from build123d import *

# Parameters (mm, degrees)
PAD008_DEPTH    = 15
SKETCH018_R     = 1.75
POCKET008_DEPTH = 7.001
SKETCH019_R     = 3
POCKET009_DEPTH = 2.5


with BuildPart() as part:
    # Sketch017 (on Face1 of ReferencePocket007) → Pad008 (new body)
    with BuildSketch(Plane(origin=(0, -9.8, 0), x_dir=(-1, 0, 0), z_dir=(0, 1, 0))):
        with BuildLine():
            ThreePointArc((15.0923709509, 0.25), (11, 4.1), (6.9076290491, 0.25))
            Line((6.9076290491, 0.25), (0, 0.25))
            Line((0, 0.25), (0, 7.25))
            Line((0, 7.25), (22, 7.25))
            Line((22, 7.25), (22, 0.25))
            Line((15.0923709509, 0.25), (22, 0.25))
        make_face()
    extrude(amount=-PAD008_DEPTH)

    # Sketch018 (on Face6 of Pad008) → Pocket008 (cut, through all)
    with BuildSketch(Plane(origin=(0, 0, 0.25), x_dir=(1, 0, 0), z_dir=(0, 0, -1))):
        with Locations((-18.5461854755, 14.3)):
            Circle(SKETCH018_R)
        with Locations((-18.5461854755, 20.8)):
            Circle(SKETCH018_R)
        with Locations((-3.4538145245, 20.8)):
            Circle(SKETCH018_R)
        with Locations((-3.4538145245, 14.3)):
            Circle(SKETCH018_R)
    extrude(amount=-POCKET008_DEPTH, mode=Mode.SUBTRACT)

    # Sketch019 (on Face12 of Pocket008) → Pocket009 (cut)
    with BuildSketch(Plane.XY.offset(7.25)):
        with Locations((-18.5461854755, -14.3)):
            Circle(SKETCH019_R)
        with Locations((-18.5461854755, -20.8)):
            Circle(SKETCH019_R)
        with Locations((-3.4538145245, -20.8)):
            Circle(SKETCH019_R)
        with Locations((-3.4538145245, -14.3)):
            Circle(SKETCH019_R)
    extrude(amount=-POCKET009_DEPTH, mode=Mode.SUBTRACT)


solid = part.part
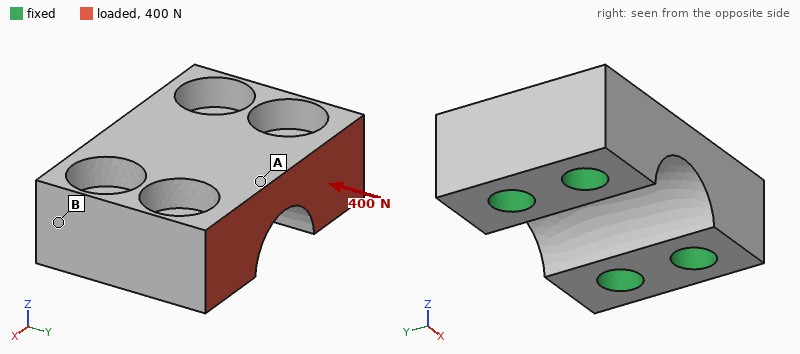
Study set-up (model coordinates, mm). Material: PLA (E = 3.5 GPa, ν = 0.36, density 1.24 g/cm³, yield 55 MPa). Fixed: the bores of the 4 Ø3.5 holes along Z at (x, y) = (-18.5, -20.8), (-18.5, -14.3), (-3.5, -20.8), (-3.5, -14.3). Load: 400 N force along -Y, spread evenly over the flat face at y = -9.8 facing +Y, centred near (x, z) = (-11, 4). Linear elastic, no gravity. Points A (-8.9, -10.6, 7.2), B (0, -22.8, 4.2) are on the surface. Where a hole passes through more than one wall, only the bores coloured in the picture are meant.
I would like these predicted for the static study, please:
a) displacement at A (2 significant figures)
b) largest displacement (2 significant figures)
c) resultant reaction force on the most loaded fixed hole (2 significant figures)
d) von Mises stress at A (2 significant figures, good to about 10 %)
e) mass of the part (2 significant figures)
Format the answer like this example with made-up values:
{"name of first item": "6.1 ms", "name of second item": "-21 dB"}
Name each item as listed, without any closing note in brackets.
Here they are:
{"displacement at A": "16 µm", "largest displacement": "24 µm", "resultant reaction force on the most loaded fixed hole": "160 N", "von Mises stress at A": "3.4 MPa", "mass of the part": "1.8 g"}
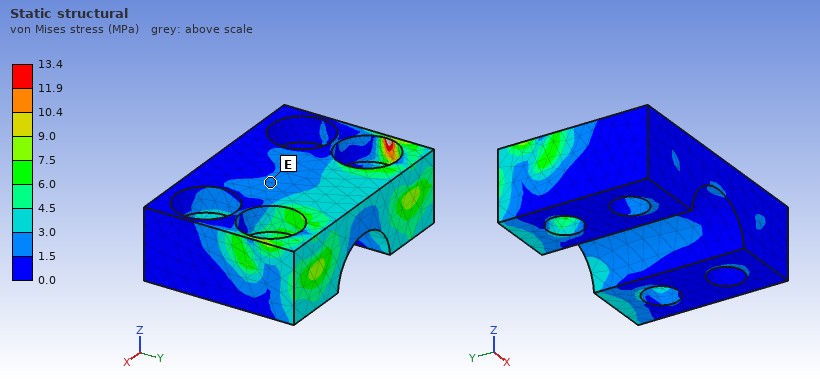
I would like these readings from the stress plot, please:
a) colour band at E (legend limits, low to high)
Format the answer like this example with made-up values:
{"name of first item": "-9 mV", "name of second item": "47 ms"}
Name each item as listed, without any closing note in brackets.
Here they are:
{"colour band at E": "1.5 to 3.0 MPa"}
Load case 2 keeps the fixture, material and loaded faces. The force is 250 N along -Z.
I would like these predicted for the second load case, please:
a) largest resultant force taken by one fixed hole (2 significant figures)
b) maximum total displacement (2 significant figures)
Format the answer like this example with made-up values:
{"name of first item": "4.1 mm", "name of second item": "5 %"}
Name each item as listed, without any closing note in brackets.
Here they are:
{"largest resultant force taken by one fixed hole": "140 N", "maximum total displacement": "30 µm"}
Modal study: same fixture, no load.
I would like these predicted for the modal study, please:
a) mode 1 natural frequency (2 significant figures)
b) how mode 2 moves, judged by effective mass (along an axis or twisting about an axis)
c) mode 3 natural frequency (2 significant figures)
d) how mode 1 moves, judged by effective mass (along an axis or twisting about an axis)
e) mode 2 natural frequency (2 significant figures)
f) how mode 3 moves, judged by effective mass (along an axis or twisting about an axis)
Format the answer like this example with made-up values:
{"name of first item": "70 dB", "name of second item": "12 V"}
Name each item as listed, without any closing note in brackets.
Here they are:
{"mode 1 natural frequency": "25 kHz", "how mode 2 moves, judged by effective mass": "along Z", "mode 3 natural frequency": "37 kHz", "how mode 1 moves, judged by effective mass": "along Y", "mode 2 natural frequency": "31 kHz", "how mode 3 moves, judged by effective mass": "along X"}
